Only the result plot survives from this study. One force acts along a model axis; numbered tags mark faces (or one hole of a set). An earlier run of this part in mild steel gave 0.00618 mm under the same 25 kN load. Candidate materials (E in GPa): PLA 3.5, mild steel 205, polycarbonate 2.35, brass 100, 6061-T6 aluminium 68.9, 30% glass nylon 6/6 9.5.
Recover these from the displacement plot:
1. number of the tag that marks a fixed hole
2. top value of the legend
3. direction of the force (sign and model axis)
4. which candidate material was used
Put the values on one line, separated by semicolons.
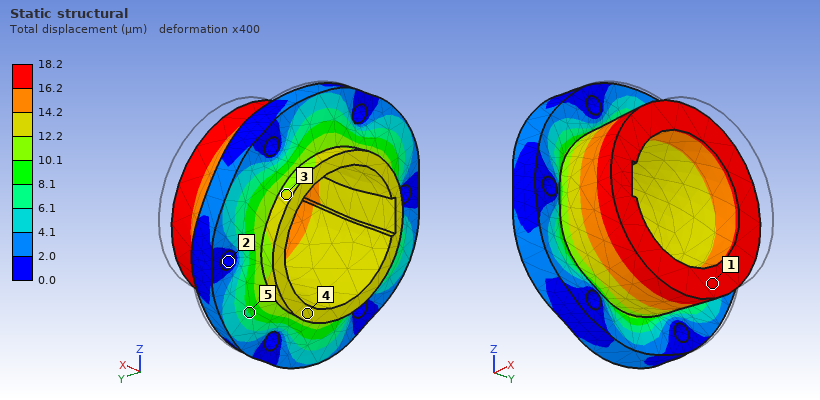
2; 18.2 µm; -X; 6061-T6 aluminium
